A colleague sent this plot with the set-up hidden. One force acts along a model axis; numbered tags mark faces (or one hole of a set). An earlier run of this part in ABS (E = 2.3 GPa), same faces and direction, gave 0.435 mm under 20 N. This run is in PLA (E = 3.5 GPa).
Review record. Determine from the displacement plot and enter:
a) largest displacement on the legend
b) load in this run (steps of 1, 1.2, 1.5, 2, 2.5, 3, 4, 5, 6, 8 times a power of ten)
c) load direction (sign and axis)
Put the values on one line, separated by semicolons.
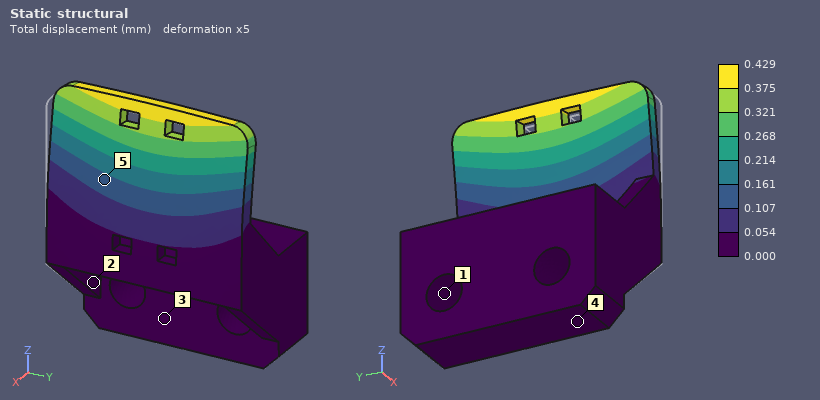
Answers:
0.429 mm; 30 N; -X
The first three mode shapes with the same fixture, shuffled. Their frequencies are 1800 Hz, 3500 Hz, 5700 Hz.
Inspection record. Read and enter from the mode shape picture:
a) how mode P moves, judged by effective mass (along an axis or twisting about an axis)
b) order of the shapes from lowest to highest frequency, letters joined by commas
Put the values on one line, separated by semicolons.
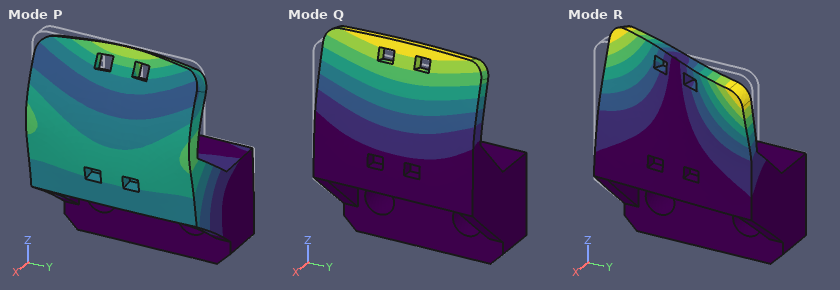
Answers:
along Z; Q, R, P
